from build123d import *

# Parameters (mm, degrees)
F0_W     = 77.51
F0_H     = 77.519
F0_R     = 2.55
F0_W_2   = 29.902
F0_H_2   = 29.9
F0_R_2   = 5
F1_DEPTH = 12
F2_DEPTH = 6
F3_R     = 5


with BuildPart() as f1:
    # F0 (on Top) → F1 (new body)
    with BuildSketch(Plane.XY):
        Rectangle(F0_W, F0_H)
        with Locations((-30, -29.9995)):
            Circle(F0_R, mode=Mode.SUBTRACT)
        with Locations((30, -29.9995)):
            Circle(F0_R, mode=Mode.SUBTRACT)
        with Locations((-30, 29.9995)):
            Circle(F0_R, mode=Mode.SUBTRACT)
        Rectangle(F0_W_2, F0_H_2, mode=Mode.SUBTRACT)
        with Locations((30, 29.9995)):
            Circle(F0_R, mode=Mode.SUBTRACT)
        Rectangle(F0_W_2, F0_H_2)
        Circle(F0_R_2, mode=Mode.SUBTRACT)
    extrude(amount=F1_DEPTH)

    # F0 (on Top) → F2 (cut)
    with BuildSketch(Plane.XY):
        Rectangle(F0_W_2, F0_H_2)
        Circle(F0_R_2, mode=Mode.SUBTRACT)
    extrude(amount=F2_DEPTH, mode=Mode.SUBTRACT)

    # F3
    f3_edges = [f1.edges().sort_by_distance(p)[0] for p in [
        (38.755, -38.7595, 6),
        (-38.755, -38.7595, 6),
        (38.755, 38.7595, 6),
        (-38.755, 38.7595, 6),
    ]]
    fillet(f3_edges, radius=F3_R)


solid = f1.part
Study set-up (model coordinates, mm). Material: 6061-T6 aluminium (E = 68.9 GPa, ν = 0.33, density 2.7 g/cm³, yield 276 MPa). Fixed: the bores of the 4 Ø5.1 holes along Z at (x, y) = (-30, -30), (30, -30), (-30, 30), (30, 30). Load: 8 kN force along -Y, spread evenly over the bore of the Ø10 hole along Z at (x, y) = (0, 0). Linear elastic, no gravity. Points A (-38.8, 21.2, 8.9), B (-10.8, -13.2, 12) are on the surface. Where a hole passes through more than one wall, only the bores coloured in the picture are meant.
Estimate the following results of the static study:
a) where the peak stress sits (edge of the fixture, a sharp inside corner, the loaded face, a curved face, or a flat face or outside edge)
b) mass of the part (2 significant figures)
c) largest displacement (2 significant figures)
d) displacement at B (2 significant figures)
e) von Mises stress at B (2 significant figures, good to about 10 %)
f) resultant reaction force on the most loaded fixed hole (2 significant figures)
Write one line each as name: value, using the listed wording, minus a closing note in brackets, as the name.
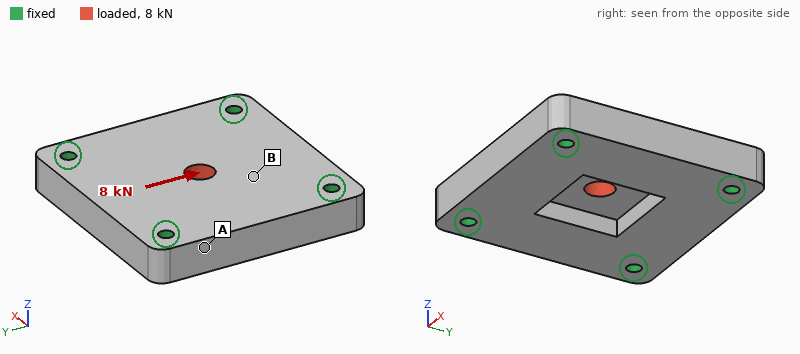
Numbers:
where the peak stress sits: the loaded face
mass of the part: 180 g
largest displacement: 12 µm
displacement at B: 6.1 µm
von Mises stress at B: 18 MPa
resultant reaction force on the most loaded fixed hole: 2.2 kN
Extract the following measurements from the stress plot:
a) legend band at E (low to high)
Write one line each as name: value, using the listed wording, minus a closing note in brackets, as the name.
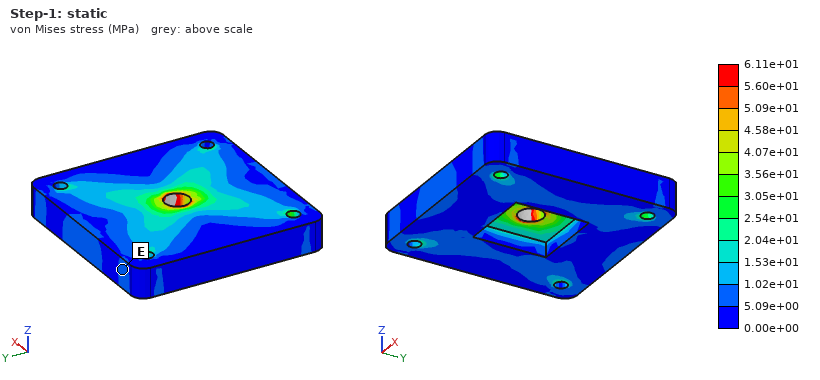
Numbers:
legend band at E: 5.09e+00 to 1.02e+01 MPa
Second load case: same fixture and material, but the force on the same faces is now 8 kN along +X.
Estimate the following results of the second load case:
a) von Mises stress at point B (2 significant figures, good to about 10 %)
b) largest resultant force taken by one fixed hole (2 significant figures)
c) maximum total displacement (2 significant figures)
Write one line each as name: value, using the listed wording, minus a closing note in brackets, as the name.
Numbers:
von Mises stress at point B: 17 MPa
largest resultant force taken by one fixed hole: 2.2 kN
maximum total displacement: 12 µm
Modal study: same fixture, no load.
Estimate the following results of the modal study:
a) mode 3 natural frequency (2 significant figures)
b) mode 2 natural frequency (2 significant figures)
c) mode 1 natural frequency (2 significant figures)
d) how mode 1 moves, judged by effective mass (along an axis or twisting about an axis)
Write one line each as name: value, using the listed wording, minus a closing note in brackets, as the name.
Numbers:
mode 3 natural frequency: 14 kHz
mode 2 natural frequency: 14 kHz
mode 1 natural frequency: 9800 Hz
how mode 1 moves, judged by effective mass: along Z
